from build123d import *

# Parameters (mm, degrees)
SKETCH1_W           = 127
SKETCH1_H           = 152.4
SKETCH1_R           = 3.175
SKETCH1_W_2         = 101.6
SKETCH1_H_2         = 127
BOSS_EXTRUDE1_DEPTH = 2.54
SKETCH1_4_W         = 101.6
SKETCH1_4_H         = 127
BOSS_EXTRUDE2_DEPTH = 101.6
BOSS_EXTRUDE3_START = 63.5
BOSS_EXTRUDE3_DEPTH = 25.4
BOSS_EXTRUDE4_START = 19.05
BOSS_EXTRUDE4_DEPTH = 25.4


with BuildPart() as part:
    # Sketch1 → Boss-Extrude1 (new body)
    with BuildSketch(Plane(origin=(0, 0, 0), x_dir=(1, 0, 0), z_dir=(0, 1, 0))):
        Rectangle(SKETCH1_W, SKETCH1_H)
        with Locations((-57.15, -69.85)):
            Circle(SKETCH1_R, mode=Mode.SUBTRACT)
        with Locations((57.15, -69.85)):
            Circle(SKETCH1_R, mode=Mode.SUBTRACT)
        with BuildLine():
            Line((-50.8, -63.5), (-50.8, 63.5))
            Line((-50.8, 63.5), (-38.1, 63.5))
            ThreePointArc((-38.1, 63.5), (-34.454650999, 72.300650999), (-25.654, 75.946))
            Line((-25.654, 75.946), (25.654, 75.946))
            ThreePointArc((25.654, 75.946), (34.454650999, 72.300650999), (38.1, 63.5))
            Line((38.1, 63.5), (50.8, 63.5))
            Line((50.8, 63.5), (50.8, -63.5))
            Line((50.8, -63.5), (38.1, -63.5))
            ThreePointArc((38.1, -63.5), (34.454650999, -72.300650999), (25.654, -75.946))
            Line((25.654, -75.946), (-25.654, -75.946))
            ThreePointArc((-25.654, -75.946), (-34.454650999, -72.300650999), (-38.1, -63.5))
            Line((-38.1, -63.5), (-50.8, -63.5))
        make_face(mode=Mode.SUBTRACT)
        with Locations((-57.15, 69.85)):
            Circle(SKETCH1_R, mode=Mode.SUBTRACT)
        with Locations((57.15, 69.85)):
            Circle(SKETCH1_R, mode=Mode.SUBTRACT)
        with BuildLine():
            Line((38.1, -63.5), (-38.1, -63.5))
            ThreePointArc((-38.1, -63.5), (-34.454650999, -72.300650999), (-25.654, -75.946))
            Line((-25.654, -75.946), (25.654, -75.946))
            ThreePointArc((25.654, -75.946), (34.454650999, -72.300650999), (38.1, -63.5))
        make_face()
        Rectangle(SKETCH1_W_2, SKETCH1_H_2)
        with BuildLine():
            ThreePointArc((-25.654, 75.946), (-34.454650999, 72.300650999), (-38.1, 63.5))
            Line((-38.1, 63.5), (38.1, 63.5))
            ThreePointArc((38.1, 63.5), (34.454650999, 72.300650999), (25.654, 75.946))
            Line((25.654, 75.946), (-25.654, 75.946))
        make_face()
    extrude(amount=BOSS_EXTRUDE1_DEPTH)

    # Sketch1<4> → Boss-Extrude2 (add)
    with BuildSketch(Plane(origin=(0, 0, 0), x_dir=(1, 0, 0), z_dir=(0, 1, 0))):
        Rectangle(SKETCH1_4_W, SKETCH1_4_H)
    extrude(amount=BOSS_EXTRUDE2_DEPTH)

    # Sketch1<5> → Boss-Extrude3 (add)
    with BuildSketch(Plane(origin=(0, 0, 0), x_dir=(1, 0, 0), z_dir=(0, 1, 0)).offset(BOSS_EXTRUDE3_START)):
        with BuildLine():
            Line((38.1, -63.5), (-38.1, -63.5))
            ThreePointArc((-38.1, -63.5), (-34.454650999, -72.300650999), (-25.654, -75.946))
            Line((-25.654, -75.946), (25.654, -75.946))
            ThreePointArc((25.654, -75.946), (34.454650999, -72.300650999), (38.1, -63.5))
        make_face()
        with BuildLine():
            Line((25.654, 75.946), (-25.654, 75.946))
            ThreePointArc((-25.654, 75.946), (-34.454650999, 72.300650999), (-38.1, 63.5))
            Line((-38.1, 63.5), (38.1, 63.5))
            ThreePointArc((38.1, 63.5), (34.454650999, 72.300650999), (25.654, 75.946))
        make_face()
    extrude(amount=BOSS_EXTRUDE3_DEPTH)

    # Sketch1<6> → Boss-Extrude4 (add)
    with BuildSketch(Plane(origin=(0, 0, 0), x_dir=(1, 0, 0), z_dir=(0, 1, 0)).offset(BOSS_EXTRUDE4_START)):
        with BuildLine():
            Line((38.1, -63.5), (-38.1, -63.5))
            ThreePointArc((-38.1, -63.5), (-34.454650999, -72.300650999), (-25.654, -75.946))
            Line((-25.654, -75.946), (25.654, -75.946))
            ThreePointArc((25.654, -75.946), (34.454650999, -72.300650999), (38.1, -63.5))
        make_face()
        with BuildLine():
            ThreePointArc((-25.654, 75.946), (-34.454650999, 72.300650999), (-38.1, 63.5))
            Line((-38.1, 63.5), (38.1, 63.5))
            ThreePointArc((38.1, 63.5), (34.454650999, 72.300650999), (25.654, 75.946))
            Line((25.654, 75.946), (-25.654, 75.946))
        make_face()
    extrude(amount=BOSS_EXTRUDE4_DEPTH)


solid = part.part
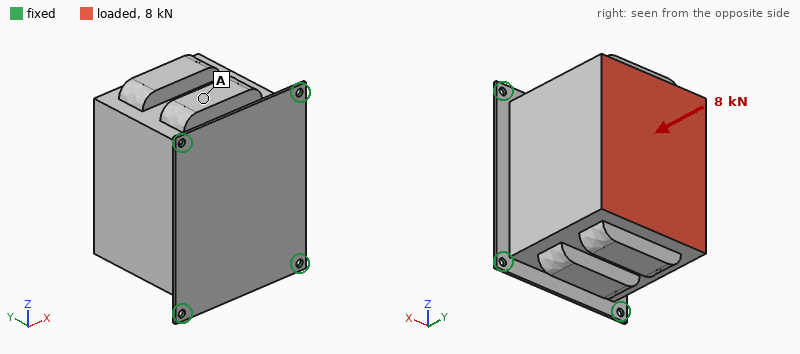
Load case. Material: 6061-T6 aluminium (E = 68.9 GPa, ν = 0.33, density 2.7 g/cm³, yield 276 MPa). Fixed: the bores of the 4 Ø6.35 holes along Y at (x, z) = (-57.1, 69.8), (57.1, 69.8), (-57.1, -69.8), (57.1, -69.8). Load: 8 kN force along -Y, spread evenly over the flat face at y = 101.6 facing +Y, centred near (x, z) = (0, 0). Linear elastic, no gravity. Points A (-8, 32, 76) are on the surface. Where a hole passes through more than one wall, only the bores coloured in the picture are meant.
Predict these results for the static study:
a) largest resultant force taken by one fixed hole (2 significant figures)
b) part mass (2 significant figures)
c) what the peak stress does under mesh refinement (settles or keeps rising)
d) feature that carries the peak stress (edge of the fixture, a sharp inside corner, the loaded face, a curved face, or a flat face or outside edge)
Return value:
2.3 kN
3.8 kg
keeps rising
edge of the fixture
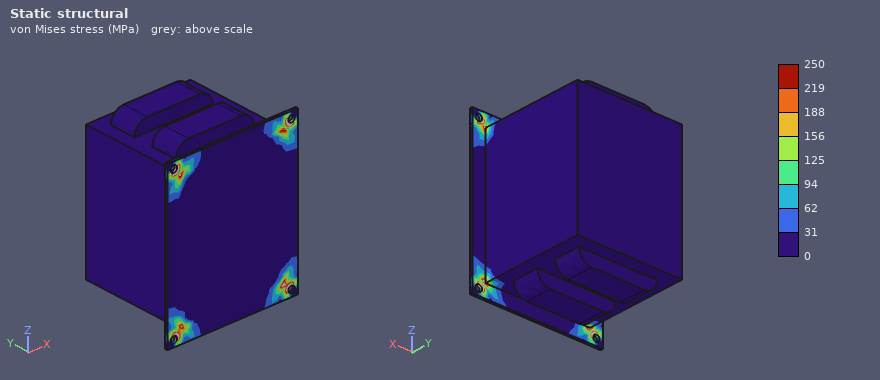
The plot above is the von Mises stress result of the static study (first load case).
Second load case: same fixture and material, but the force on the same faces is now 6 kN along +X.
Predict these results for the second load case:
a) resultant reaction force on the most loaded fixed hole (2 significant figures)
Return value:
3.5 kN
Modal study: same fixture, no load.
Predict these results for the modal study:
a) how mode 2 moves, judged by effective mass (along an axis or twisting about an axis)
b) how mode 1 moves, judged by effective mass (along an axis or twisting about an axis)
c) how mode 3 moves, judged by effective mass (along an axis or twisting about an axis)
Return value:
along Z
along X
along Y
